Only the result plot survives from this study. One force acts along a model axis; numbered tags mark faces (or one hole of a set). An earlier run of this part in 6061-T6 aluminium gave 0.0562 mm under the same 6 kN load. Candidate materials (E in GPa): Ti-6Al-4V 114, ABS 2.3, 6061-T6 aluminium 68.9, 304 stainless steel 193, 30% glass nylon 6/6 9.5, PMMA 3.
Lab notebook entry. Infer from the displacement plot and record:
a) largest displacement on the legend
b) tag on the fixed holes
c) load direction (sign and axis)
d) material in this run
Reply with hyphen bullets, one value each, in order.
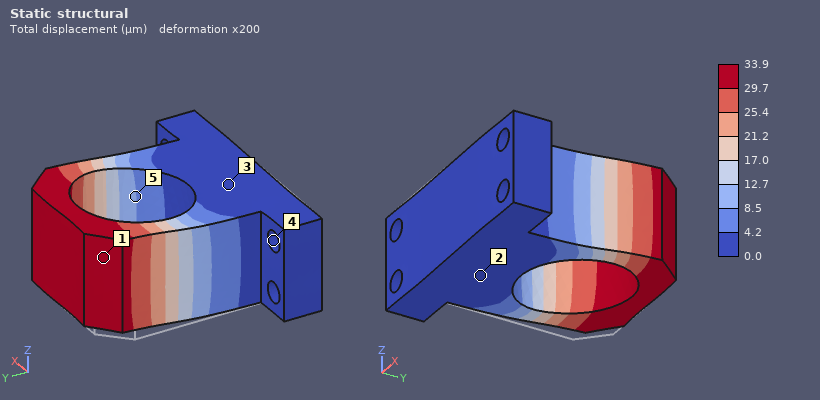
- 33.9 µm
- 4
- +X
- Ti-6Al-4V
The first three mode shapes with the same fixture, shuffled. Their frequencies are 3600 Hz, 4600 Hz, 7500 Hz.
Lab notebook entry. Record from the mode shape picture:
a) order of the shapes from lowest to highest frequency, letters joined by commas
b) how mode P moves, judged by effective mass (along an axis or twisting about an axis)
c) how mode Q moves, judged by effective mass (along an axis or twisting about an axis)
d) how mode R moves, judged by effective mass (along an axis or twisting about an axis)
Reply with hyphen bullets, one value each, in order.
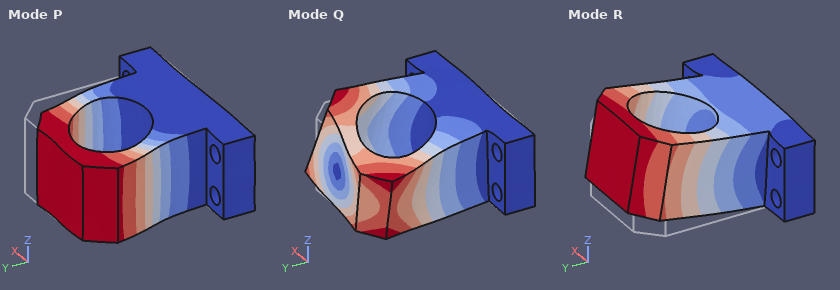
- R, P, Q
- along X
- twisting about Y
- along Z
